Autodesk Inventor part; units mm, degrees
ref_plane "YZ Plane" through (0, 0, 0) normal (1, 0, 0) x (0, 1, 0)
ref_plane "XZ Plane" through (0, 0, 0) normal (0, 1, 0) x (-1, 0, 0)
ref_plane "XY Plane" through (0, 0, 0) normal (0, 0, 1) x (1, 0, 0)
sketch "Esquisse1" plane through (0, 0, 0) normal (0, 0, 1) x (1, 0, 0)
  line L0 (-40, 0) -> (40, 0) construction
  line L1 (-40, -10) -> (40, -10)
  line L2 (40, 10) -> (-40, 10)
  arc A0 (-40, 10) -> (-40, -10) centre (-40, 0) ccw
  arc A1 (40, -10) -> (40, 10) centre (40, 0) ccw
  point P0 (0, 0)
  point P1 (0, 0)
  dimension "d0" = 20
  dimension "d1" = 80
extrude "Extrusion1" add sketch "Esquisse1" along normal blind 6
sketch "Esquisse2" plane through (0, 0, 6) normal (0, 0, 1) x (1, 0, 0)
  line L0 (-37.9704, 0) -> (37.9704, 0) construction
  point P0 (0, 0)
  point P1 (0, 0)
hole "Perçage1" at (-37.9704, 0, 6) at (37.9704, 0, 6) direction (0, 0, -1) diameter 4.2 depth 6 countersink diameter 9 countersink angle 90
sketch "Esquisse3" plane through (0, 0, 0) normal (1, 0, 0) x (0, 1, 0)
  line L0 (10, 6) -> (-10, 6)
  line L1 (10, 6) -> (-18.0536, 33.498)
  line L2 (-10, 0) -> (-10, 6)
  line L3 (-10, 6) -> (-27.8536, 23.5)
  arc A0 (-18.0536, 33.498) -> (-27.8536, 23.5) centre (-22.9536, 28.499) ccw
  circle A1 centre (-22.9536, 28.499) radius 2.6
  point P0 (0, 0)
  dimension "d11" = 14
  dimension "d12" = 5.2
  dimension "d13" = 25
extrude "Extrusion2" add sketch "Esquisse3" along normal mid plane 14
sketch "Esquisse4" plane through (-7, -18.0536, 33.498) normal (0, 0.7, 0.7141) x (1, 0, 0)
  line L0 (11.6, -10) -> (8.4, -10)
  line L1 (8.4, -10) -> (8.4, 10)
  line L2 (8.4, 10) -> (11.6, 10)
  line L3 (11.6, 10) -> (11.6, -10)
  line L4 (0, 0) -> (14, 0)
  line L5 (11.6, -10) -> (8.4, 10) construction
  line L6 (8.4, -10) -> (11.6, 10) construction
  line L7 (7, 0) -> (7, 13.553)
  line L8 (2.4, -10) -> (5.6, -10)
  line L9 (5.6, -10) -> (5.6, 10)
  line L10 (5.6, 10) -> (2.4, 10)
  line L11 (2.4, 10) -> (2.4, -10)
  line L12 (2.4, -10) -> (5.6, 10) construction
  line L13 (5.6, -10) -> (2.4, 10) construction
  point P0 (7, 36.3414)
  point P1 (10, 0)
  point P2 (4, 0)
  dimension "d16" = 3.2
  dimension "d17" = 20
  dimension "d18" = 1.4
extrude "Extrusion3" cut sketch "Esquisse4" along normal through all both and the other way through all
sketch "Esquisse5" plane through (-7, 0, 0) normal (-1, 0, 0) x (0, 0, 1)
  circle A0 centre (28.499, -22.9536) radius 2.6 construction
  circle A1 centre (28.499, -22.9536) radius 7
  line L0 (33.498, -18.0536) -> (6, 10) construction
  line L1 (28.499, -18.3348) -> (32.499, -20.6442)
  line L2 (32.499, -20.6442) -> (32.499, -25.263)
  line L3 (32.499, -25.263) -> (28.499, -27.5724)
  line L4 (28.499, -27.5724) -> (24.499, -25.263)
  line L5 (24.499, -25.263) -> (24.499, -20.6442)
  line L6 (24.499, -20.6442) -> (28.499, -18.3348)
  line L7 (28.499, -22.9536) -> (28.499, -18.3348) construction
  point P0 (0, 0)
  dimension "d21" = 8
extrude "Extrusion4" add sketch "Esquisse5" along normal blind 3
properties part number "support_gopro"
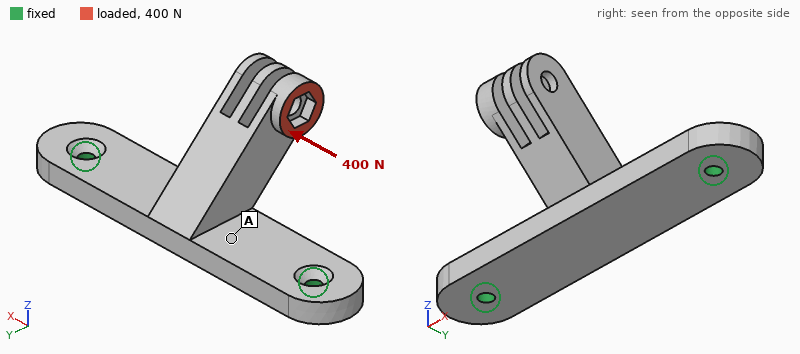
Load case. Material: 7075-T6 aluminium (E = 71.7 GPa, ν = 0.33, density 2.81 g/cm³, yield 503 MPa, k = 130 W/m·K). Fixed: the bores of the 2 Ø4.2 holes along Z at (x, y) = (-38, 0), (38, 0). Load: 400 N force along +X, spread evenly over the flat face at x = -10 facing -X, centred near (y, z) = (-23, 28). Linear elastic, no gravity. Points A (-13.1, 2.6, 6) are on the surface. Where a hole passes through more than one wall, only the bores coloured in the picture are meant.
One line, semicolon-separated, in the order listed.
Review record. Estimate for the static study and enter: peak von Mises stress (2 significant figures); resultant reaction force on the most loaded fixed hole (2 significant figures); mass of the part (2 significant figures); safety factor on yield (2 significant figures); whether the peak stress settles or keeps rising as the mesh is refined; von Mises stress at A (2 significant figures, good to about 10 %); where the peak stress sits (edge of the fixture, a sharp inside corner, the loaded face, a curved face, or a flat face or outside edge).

250 MPa; 300 N; 49 g; 2.0; settles; 21 MPa; a flat face or outside edge
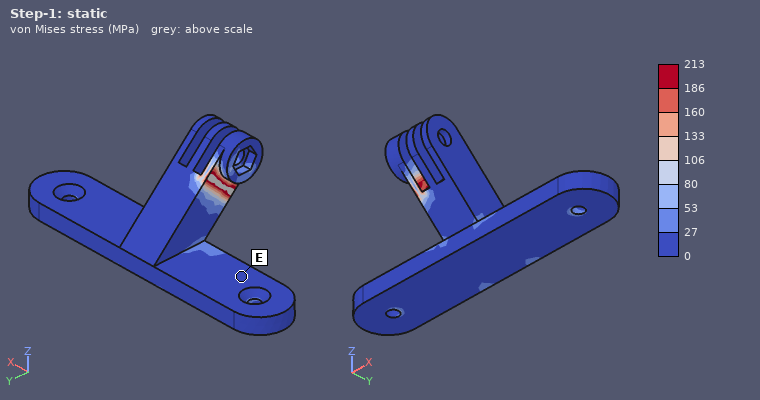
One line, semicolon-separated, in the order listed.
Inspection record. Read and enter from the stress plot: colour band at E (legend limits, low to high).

0 to 27 MPa
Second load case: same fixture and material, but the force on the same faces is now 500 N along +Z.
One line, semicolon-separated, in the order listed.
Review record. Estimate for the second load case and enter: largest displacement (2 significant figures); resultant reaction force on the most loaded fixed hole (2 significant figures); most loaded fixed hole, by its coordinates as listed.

0.39 mm; 460 N; (-38, 0)
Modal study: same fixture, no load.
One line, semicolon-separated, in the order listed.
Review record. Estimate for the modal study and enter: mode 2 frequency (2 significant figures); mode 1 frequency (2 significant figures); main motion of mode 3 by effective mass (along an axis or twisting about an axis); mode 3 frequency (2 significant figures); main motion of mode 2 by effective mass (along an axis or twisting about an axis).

3500 Hz; 2100 Hz; along X; 4200 Hz; along Z
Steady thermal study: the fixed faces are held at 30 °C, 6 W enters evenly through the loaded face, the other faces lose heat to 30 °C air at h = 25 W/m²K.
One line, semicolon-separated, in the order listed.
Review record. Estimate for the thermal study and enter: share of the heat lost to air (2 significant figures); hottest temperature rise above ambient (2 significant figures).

19 %; 26 K
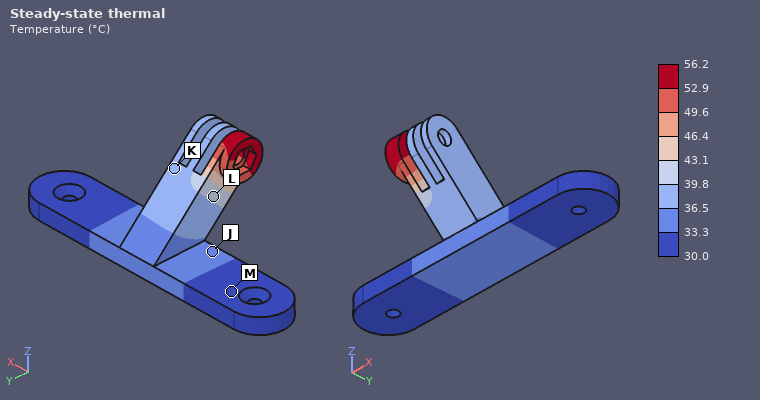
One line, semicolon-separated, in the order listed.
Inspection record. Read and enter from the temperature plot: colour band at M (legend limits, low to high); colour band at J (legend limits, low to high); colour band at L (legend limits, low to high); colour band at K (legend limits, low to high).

30.0 to 33.3 °C; 33.3 to 36.5 °C; 39.8 to 43.1 °C; 36.5 to 39.8 °C
